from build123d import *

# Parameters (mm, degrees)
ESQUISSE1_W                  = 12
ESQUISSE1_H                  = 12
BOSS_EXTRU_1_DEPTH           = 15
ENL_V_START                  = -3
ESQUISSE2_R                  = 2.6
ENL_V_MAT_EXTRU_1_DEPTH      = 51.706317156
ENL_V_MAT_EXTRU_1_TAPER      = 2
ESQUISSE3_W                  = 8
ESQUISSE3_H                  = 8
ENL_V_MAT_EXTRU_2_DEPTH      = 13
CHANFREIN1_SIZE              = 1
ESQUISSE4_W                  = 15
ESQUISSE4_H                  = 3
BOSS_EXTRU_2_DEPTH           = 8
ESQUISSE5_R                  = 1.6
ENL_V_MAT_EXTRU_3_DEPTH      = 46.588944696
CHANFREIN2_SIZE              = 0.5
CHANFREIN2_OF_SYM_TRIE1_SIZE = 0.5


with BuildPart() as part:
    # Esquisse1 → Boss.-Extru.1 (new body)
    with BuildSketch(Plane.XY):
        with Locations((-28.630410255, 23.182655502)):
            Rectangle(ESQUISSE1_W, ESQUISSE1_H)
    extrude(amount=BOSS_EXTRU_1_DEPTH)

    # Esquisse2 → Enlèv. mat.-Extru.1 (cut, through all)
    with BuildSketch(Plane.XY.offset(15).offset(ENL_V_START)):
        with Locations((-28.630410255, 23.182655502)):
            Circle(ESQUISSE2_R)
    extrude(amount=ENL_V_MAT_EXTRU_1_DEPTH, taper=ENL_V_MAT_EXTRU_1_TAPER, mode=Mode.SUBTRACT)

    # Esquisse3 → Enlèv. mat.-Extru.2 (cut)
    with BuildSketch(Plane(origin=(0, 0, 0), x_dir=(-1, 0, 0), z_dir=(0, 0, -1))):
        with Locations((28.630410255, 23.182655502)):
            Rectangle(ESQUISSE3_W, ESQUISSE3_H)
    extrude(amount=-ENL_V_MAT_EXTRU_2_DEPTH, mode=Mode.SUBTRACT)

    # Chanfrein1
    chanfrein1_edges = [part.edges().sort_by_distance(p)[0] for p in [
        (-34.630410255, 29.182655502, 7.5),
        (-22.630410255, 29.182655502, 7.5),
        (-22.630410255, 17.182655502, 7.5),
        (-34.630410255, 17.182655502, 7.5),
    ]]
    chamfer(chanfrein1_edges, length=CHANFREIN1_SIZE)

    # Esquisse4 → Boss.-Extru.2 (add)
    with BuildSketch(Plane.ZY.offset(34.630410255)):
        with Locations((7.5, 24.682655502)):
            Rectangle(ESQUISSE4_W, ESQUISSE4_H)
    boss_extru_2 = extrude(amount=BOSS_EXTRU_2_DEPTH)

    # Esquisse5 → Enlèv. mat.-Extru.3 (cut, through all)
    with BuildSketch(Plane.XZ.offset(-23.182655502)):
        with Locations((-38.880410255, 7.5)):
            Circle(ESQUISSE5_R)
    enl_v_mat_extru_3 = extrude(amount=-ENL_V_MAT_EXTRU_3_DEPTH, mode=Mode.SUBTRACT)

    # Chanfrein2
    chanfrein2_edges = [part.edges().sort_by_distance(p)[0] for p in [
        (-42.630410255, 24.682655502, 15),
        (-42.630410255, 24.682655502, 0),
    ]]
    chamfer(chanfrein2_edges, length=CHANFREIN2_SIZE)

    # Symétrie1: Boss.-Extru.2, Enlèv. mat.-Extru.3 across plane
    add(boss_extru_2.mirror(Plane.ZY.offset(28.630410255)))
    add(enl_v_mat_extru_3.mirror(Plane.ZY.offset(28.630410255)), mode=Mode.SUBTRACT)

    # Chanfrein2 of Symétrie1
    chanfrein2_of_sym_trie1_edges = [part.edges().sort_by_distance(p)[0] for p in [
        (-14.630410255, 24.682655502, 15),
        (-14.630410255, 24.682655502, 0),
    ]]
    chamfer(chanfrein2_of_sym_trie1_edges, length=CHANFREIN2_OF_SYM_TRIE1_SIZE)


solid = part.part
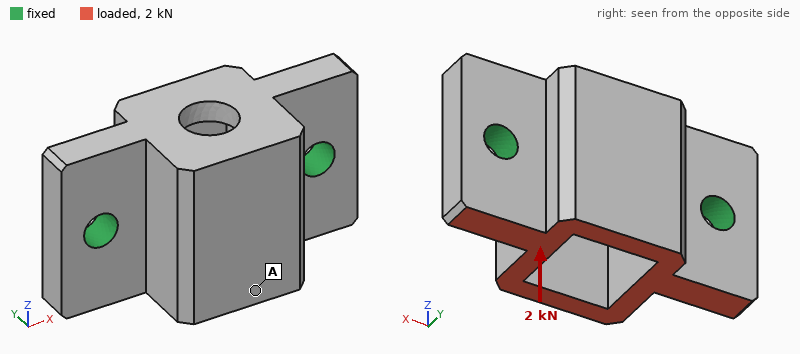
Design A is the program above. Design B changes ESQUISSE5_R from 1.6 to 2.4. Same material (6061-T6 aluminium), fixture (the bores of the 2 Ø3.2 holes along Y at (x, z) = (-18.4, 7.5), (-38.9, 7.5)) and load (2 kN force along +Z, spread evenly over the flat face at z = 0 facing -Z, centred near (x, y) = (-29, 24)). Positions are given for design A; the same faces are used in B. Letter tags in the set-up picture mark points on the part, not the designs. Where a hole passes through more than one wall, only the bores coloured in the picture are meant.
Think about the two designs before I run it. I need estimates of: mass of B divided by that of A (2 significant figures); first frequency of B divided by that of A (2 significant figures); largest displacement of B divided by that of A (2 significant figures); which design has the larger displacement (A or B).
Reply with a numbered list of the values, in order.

1. 0.97
2. 1.3
3. 0.73
4. A
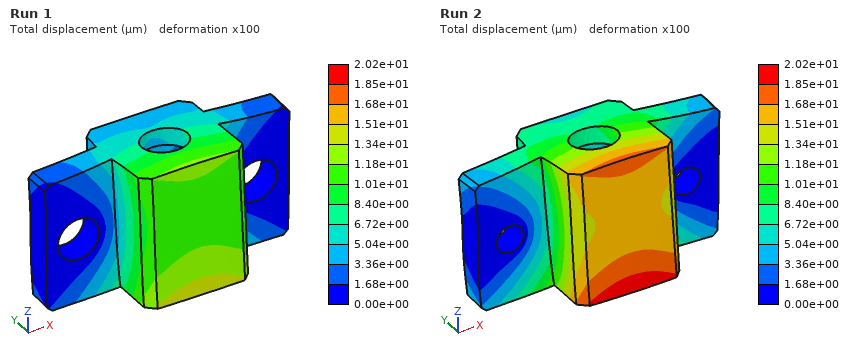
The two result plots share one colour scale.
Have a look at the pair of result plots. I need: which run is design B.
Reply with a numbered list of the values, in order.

1. Run 1
